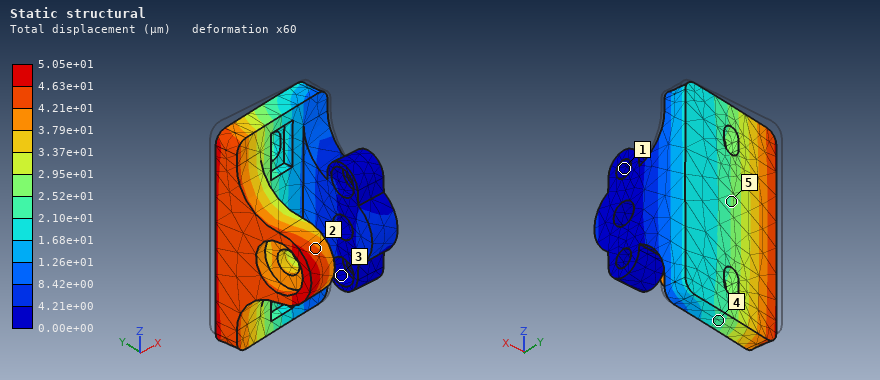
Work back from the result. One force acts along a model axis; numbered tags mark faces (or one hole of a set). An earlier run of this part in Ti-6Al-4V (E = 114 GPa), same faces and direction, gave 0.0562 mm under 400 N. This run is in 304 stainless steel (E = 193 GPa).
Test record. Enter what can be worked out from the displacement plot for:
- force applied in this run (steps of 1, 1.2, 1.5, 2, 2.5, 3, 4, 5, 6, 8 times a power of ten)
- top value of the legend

600 N
5.05e+01 µm
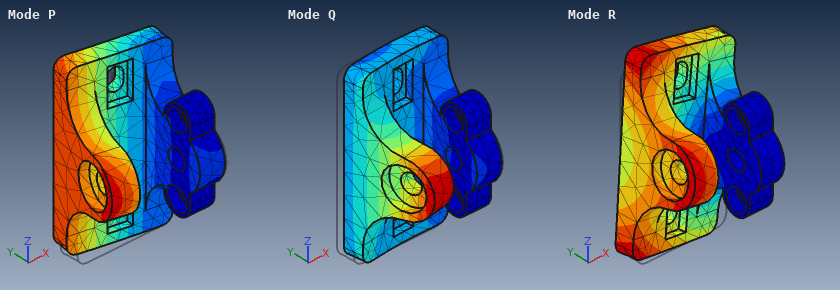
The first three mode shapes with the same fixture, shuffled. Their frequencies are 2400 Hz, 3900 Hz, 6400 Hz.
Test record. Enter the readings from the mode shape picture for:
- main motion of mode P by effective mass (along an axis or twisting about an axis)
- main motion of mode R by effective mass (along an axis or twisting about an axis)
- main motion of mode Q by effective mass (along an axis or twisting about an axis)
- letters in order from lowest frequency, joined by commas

along Y
along Z
along X
P, R, Q
